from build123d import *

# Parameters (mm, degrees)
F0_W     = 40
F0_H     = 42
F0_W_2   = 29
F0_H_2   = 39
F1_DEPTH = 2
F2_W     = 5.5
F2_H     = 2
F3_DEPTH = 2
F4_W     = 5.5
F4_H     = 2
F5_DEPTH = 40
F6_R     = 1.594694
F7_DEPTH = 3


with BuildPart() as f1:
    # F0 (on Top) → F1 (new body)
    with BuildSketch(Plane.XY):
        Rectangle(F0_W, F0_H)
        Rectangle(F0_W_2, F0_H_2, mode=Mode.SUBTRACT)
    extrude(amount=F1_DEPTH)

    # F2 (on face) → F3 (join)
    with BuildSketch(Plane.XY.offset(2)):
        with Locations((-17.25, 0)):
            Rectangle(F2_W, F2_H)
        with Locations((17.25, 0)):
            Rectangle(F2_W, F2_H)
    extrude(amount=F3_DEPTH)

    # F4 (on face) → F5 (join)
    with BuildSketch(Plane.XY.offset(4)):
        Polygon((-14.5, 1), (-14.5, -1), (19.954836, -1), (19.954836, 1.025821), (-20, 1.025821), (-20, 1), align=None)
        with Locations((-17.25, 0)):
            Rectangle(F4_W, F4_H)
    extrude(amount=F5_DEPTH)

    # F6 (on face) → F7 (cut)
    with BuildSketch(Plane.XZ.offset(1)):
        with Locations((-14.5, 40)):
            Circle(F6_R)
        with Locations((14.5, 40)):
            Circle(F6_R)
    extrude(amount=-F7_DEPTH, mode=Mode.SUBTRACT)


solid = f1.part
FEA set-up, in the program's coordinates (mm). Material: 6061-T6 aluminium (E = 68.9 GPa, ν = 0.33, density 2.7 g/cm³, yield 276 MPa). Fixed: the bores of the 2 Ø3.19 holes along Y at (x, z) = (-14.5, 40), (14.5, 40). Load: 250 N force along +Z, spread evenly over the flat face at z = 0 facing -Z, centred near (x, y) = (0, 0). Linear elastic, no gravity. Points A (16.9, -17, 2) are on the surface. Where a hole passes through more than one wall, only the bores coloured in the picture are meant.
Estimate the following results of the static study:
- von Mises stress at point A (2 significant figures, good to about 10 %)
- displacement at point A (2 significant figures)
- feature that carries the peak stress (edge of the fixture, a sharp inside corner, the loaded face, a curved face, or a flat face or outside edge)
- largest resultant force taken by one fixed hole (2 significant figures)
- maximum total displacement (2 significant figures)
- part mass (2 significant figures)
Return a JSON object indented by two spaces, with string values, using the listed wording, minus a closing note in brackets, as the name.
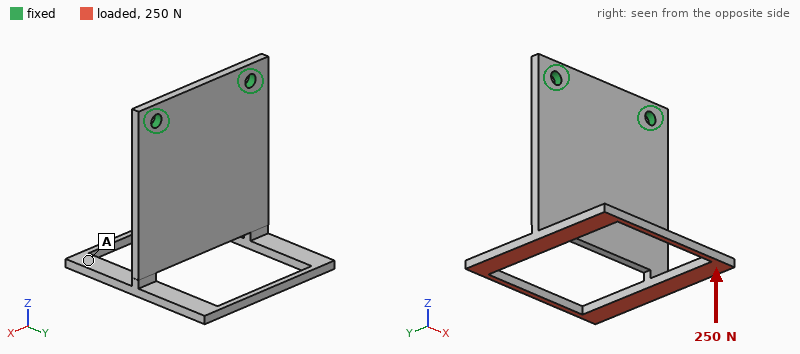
{
  "von Mises stress at point A": "21 MPa",
  "displacement at point A": "0.25 mm",
  "feature that carries the peak stress": "the loaded face",
  "largest resultant force taken by one fixed hole": "130 N",
  "maximum total displacement": "0.40 mm",
  "part mass": "12 g"
}
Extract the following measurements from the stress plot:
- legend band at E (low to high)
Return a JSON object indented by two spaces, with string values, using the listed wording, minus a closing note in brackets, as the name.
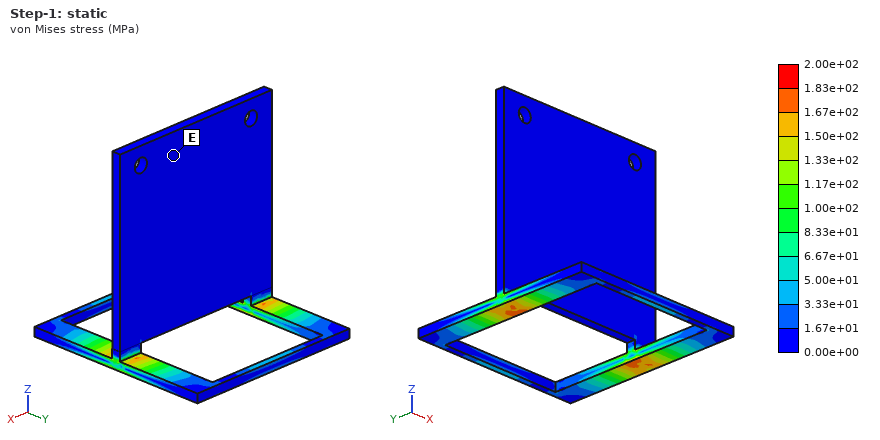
{
  "legend band at E": "0.00e+00 to 1.67e+01 MPa"
}
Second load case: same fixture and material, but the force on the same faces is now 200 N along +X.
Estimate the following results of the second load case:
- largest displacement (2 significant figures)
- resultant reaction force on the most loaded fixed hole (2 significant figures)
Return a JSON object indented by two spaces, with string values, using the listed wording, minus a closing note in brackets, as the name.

{
  "largest displacement": "61 µm",
  "resultant reaction force on the most loaded fixed hole": "280 N"
}
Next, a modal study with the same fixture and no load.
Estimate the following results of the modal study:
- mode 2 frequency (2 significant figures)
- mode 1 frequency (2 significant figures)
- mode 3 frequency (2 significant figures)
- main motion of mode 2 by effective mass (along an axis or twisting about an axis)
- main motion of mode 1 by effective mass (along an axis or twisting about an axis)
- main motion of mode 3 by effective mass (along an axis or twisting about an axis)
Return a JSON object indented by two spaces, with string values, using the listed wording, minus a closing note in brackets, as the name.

{
  "mode 2 frequency": "1200 Hz",
  "mode 1 frequency": "640 Hz",
  "mode 3 frequency": "1700 Hz",
  "main motion of mode 2 by effective mass": "twisting about Z",
  "main motion of mode 1 by effective mass": "along Y",
  "main motion of mode 3 by effective mass": "along Y"
}
